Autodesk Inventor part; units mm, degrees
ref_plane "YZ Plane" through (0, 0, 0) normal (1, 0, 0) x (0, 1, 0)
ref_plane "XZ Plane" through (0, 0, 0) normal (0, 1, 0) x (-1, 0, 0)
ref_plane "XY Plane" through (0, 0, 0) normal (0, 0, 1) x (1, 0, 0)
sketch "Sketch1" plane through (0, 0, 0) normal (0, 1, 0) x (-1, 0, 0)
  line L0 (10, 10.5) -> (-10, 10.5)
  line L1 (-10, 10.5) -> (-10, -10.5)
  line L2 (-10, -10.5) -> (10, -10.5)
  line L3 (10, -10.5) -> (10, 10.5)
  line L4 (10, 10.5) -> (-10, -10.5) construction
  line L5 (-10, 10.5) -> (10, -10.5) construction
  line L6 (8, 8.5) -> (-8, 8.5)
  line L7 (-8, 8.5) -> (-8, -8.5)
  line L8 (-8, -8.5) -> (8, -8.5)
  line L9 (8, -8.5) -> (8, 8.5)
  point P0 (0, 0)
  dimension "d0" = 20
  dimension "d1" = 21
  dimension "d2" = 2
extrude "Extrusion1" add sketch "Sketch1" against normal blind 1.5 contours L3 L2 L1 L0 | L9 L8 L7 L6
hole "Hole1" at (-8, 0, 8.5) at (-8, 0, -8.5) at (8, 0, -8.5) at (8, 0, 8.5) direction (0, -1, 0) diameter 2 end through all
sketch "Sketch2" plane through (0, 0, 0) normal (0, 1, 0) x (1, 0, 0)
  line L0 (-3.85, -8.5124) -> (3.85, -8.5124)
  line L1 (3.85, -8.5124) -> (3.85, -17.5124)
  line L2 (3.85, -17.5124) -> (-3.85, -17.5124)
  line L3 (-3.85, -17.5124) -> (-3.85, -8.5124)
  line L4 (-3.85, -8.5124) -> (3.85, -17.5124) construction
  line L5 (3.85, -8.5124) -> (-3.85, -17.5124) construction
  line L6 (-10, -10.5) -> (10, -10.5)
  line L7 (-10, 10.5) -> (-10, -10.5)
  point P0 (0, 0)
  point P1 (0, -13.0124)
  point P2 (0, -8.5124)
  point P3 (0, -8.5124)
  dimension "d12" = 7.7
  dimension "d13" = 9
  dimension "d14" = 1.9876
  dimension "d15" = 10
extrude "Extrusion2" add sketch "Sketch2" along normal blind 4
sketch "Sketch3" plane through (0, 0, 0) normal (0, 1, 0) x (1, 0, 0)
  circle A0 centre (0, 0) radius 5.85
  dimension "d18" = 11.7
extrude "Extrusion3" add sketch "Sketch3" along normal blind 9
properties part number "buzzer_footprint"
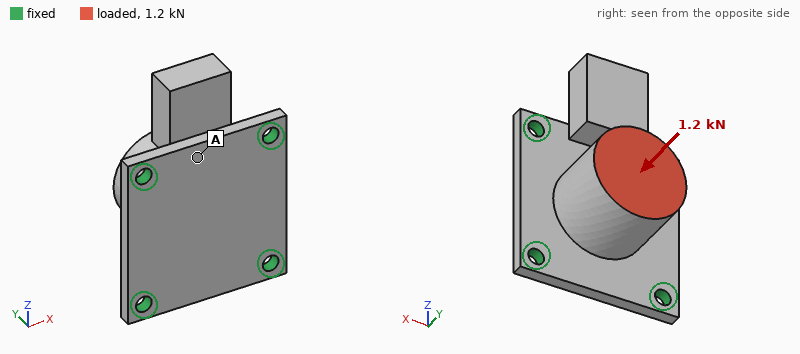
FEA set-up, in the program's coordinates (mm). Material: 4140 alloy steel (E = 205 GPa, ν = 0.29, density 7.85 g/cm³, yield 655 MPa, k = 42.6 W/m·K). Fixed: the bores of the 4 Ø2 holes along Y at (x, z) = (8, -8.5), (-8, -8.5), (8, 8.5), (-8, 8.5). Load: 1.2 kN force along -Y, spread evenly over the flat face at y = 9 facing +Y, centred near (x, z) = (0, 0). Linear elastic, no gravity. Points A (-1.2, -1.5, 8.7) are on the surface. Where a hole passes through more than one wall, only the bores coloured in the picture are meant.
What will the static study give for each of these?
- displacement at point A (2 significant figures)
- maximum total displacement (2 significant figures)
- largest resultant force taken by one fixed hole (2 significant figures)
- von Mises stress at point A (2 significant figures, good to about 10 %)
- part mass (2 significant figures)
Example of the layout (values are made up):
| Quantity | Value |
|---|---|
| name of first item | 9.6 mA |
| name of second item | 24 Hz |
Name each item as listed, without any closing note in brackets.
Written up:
| Quantity | Value |
|---|---|
| displacement at point A | 6.8 µm |
| maximum total displacement | 18 µm |
| largest resultant force taken by one fixed hole | 320 N |
| von Mises stress at point A | 48 MPa |
| part mass | 15 g |
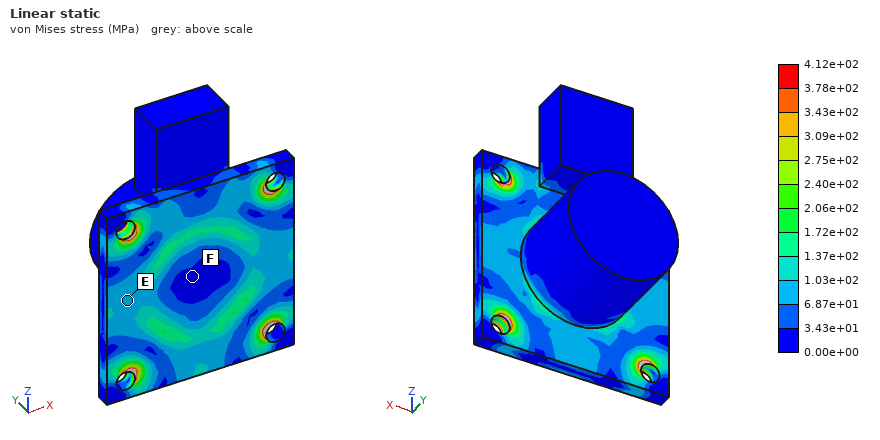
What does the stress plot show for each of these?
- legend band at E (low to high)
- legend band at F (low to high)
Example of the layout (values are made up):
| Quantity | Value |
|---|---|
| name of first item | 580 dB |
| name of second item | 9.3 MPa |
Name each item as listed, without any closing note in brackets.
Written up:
| Quantity | Value |
|---|---|
| legend band at E | 6.87e+01 to 1.03e+02 MPa |
| legend band at F | 0.00e+00 to 3.43e+01 MPa |
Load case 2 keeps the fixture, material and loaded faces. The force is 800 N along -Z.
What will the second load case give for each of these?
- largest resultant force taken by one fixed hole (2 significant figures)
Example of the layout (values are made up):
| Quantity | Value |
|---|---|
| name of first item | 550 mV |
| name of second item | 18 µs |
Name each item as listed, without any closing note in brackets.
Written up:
| Quantity | Value |
|---|---|
| largest resultant force taken by one fixed hole | 360 N |
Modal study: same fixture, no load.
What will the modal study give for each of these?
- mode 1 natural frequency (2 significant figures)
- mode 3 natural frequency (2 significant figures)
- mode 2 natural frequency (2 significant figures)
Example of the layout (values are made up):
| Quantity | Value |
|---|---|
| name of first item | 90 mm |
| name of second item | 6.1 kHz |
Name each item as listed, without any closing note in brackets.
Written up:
| Quantity | Value |
|---|---|
| mode 1 natural frequency | 8000 Hz |
| mode 3 natural frequency | 14 kHz |
| mode 2 natural frequency | 14 kHz |
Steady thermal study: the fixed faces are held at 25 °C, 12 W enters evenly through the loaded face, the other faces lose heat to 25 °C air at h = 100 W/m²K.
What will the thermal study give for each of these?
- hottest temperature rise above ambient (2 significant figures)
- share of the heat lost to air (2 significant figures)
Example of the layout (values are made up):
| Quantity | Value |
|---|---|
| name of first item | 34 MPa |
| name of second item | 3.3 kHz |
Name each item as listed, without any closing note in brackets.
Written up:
| Quantity | Value |
|---|---|
| hottest temperature rise above ambient | 54 K |
| share of the heat lost to air | 26 % |
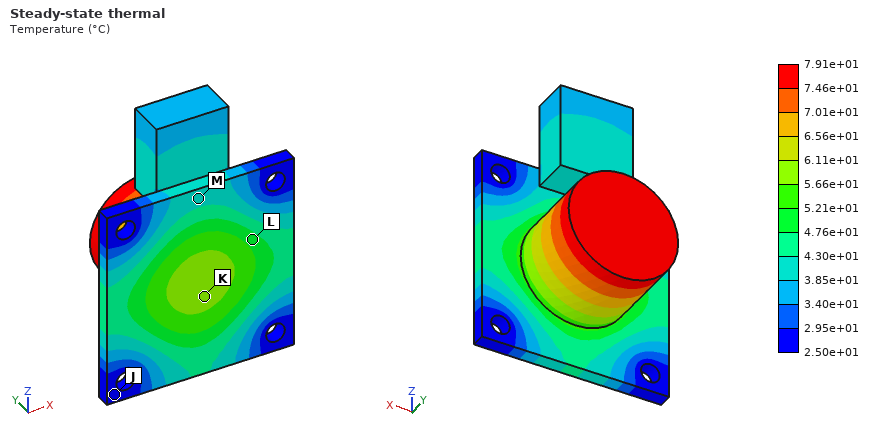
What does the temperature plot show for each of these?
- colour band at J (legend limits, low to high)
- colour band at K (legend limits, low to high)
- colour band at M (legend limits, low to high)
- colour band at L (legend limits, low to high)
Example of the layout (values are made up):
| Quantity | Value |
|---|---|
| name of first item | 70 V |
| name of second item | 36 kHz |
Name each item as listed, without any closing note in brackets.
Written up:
| Quantity | Value |
|---|---|
| colour band at J | 2.50e+01 to 2.95e+01 °C |
| colour band at K | 5.66e+01 to 6.11e+01 °C |
| colour band at M | 3.85e+01 to 4.30e+01 °C |
| colour band at L | 4.76e+01 to 5.21e+01 °C |
